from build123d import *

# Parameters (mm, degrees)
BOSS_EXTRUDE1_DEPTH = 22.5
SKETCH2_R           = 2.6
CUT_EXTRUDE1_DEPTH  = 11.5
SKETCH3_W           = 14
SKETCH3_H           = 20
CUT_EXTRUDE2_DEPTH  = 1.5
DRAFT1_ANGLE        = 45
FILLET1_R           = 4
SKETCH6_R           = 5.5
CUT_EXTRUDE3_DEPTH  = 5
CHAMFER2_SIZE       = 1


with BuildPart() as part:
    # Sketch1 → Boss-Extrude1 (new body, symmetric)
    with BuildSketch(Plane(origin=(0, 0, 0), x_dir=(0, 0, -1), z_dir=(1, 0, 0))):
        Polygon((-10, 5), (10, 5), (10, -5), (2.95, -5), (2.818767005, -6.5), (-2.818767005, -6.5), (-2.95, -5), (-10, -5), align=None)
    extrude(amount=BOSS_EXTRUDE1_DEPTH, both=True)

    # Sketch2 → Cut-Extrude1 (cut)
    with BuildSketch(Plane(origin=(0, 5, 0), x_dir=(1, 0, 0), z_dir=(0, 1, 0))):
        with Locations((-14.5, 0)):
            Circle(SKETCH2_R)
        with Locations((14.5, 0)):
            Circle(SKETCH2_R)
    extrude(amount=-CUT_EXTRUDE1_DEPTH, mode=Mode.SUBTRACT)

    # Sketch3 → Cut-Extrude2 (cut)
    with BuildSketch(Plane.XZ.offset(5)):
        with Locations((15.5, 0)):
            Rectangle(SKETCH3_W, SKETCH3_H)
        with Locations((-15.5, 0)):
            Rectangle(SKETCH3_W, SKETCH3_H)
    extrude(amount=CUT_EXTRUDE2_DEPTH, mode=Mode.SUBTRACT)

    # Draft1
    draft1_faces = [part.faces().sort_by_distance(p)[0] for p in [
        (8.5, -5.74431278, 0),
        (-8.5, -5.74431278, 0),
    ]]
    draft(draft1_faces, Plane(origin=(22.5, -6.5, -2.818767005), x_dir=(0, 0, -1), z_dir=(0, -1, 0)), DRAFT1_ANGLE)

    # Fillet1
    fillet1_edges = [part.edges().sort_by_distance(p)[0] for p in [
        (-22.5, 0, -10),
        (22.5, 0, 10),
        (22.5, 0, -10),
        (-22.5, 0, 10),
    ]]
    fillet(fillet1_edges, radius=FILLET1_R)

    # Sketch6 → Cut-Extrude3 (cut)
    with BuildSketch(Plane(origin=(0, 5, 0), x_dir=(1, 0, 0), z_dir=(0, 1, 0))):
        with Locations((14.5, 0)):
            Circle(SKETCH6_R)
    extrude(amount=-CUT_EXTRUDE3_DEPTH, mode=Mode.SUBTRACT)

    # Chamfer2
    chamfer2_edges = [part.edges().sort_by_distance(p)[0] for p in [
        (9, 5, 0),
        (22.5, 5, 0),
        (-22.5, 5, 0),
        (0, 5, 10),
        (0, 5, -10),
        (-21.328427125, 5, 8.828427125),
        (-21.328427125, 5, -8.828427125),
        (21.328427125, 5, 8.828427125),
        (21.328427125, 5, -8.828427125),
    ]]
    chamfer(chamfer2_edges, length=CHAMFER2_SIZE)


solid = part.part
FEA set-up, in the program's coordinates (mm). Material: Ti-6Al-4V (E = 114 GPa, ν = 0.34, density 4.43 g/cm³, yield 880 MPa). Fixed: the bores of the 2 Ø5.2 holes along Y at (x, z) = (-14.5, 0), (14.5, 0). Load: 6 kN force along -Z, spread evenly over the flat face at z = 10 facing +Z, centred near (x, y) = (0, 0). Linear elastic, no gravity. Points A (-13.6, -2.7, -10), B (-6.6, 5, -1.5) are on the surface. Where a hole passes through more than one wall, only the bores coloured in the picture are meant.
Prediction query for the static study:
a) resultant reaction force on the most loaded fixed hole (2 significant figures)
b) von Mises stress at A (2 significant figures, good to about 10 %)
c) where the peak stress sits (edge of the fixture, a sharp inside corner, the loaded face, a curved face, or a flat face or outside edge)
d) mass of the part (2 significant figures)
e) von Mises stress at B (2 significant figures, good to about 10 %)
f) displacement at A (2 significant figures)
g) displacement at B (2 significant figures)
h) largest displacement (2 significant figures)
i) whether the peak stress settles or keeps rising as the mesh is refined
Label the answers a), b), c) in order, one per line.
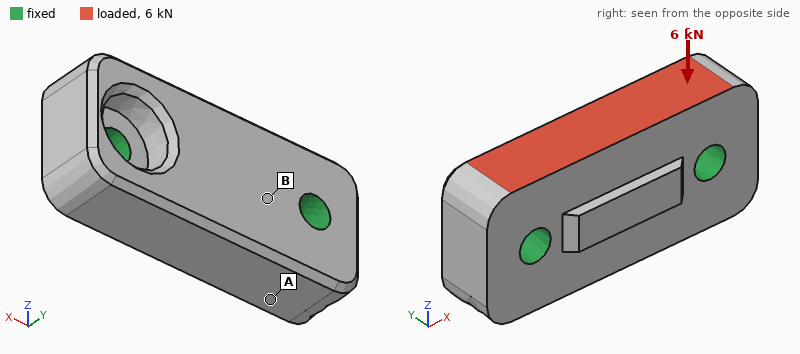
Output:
a) 3.2 kN
b) 6.9 MPa
c) edge of the fixture
d) 36 g
e) 21 MPa
f) 1.5 µm
g) 2.9 µm
h) 6.5 µm
i) keeps rising
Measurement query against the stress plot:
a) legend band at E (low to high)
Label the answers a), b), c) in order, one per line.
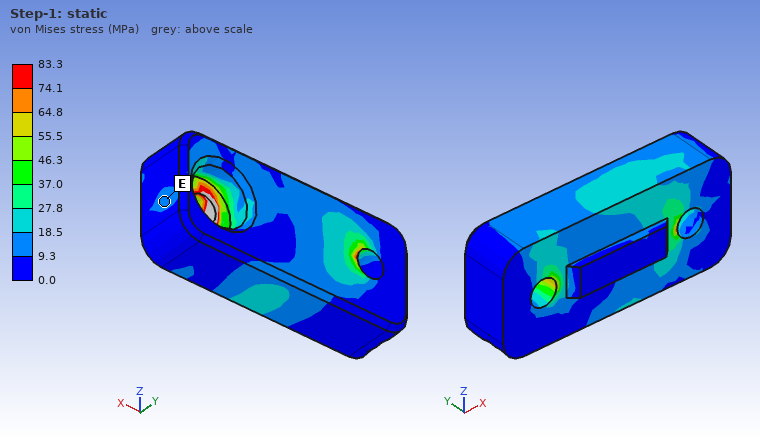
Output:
a) 9.3 to 18.5 MPa
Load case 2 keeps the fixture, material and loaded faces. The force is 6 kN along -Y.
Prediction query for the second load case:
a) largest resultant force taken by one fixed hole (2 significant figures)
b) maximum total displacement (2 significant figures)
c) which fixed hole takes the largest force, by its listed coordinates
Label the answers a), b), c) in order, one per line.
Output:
a) 3.3 kN
b) 29 µm
c) (-14.5, 0)
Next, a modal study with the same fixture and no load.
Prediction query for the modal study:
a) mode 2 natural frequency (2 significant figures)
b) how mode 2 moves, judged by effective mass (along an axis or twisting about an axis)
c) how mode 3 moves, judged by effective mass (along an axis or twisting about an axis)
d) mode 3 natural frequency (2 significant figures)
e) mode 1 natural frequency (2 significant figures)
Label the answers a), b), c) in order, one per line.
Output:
a) 32 kHz
b) along Y
c) along Z
d) 38 kHz
e) 26 kHz
